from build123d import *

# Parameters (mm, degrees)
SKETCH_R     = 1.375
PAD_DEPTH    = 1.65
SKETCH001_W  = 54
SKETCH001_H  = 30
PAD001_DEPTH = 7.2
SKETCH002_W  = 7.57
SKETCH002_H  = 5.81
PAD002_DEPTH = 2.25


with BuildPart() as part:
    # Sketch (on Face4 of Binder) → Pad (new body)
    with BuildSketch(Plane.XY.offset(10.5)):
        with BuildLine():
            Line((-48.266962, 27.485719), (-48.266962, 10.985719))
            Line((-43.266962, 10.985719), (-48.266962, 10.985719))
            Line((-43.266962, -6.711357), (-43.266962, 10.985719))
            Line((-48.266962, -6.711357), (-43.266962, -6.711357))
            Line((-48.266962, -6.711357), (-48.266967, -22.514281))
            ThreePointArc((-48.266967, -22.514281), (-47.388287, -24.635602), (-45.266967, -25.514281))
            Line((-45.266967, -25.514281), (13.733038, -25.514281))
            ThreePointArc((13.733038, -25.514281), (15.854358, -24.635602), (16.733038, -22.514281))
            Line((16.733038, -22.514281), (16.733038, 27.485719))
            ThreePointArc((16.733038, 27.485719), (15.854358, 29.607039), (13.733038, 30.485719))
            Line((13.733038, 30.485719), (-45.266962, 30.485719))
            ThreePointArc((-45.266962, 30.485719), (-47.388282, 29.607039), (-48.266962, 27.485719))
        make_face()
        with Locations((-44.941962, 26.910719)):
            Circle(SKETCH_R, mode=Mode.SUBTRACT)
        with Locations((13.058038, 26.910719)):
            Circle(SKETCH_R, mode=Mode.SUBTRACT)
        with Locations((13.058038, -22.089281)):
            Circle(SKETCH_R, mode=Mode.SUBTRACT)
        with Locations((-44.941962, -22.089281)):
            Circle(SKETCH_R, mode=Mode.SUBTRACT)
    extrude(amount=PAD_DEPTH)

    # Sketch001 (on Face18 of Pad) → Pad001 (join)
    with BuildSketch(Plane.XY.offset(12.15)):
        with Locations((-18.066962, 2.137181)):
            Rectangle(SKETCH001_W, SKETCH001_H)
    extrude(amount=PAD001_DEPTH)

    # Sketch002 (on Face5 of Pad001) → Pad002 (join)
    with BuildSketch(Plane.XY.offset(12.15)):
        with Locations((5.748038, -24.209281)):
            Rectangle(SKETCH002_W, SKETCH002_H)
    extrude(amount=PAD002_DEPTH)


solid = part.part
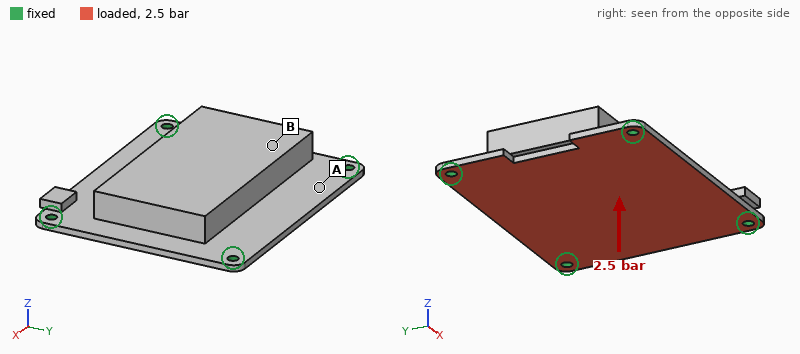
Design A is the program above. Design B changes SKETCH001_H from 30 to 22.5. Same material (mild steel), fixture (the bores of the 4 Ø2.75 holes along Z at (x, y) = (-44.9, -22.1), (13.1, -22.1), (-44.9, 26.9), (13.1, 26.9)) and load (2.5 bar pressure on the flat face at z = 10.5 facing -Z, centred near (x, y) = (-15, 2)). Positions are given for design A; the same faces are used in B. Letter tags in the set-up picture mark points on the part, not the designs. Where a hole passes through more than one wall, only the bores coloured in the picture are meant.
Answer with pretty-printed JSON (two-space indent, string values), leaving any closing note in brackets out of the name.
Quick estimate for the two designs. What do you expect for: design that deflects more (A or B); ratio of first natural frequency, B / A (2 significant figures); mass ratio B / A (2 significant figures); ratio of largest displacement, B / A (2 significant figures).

{
  "design that deflects more": "B",
  "ratio of first natural frequency, B / A": "0.82",
  "mass ratio B / A": "0.83",
  "ratio of largest displacement, B / A": "1.5"
}
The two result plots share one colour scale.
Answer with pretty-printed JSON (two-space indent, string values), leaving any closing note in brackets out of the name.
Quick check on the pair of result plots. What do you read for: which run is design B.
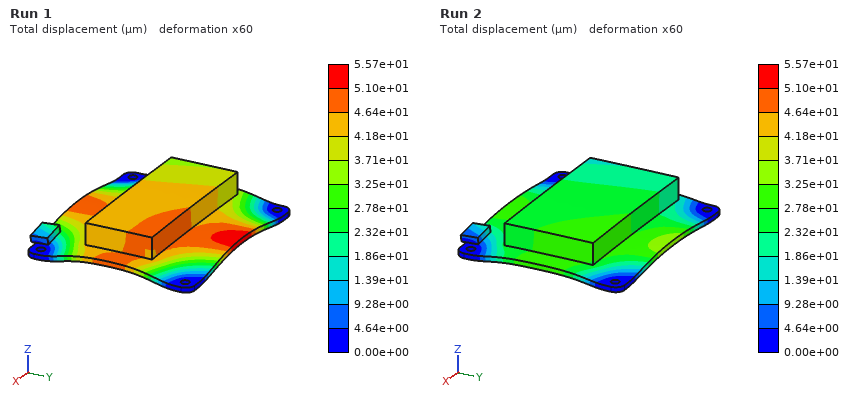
{
  "which run is design B": "Run 1"
}
